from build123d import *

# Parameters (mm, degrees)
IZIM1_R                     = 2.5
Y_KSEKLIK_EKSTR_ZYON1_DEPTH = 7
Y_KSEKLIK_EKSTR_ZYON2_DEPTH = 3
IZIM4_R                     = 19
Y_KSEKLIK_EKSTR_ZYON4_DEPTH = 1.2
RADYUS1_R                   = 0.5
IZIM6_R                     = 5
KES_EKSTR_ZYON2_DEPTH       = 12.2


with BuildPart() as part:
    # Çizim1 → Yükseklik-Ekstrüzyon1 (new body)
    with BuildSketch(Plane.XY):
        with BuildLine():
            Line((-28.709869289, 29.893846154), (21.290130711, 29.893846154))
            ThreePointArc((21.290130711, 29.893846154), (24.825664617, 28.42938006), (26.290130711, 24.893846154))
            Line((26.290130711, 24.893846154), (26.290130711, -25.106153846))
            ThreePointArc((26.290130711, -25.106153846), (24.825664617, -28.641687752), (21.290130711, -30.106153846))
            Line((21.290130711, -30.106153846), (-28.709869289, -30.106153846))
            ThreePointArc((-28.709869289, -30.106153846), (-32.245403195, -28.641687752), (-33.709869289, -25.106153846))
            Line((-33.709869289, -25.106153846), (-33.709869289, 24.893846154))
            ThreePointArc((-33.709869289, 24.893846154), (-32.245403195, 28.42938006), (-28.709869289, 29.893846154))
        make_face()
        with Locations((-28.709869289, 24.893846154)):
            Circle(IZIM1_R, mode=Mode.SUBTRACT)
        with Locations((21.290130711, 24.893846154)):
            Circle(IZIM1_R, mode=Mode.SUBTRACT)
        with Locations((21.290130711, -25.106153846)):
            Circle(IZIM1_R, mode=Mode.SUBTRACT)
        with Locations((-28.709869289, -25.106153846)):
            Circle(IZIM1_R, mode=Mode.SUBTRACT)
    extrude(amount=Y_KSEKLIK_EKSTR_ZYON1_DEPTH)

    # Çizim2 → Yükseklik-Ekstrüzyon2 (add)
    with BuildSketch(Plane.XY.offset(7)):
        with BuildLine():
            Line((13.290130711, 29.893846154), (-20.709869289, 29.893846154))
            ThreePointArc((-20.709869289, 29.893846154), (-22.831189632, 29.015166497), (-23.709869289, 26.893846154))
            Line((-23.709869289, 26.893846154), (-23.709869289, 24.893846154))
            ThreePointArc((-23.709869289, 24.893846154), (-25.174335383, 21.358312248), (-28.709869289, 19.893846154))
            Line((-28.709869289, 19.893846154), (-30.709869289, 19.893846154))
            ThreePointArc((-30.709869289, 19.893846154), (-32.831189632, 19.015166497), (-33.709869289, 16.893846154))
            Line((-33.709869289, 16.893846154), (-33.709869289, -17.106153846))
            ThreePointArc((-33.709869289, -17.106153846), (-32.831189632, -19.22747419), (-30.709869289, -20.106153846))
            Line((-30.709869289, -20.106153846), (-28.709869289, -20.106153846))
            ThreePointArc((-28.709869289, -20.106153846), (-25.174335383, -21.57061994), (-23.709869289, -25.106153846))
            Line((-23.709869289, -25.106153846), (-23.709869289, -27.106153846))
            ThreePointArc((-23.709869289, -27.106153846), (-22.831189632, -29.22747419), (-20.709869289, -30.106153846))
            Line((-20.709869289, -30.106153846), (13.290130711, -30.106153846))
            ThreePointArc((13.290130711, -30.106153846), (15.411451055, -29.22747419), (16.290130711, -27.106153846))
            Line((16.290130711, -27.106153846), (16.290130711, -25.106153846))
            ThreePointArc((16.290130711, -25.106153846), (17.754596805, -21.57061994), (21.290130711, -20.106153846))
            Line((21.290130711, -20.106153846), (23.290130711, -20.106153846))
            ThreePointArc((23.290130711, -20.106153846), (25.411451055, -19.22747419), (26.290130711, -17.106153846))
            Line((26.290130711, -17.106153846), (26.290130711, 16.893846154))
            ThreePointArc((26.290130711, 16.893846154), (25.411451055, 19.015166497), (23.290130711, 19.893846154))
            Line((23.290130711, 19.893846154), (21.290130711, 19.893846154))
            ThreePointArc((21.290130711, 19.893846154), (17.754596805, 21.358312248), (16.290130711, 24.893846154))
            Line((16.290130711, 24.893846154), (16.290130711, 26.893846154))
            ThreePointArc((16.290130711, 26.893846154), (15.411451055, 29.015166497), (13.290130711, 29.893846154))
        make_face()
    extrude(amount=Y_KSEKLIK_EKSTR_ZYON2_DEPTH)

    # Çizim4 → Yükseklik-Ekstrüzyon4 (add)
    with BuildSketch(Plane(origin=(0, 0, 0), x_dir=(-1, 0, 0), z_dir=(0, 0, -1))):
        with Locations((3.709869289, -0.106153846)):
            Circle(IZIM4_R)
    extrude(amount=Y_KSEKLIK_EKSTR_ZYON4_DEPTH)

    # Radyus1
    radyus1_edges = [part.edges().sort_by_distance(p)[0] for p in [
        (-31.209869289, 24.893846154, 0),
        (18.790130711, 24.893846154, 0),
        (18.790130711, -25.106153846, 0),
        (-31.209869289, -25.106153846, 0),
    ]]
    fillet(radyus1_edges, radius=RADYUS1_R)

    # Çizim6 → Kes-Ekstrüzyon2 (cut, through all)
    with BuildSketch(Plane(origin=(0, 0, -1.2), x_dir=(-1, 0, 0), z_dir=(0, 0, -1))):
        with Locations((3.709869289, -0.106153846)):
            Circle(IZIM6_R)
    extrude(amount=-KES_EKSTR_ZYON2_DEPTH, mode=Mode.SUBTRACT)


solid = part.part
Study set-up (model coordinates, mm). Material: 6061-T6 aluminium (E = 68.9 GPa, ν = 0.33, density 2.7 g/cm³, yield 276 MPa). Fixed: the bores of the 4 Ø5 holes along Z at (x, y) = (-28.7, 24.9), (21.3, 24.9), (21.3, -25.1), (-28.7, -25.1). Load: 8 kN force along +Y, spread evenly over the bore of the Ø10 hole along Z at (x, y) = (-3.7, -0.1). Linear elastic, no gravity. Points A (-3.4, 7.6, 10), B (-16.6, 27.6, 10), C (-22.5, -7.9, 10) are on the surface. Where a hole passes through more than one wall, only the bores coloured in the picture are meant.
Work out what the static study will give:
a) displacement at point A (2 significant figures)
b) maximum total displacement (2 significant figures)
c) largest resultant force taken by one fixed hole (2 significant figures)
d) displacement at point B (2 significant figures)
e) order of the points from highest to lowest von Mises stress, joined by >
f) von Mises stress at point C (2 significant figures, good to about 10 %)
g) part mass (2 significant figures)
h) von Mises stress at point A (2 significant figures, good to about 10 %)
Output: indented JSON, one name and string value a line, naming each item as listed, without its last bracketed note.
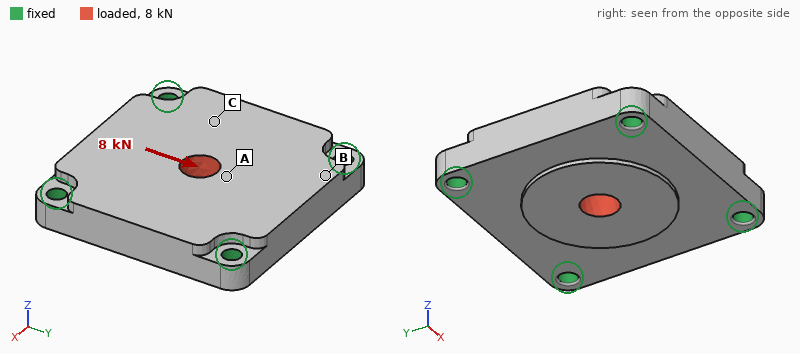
{
  "displacement at point A": "9.1 µm",
  "maximum total displacement": "10 µm",
  "largest resultant force taken by one fixed hole": "2.2 kN",
  "displacement at point B": "5.5 µm",
  "order of the points from highest to lowest von Mises stress, joined by >": "A > C > B",
  "von Mises stress at point C": "9.3 MPa",
  "part mass": "93 g",
  "von Mises stress at point A": "19 MPa"
}
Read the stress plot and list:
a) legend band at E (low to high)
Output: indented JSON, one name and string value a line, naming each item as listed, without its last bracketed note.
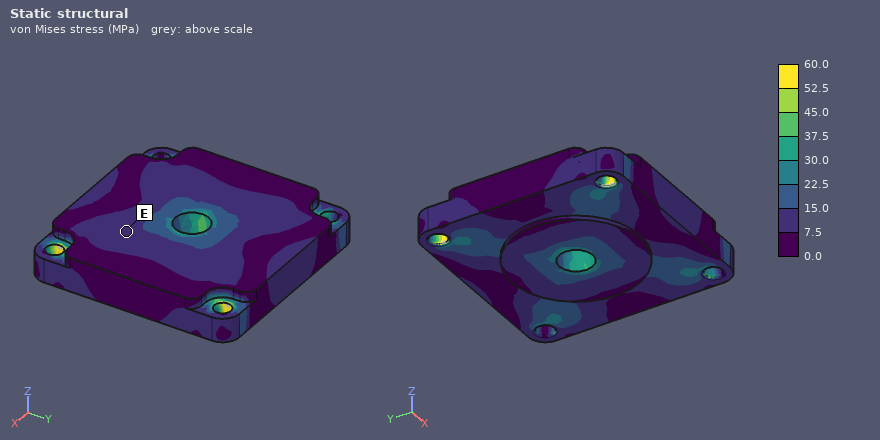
{
  "legend band at E": "7.5 to 15.0 MPa"
}
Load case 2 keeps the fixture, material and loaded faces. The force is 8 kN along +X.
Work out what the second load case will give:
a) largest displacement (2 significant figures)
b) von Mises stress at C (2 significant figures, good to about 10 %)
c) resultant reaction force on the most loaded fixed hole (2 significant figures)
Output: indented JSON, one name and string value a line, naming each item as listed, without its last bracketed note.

{
  "largest displacement": "10 µm",
  "von Mises stress at C": "8.5 MPa",
  "resultant reaction force on the most loaded fixed hole": "2.2 kN"
}
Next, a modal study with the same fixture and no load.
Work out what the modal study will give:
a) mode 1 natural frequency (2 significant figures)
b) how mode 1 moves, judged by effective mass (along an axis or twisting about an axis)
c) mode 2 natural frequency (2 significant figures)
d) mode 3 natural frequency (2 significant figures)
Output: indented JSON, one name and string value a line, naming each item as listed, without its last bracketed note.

{
  "mode 1 natural frequency": "10 kHz",
  "how mode 1 moves, judged by effective mass": "along Z",
  "mode 2 natural frequency": "16 kHz",
  "mode 3 natural frequency": "16 kHz"
}
